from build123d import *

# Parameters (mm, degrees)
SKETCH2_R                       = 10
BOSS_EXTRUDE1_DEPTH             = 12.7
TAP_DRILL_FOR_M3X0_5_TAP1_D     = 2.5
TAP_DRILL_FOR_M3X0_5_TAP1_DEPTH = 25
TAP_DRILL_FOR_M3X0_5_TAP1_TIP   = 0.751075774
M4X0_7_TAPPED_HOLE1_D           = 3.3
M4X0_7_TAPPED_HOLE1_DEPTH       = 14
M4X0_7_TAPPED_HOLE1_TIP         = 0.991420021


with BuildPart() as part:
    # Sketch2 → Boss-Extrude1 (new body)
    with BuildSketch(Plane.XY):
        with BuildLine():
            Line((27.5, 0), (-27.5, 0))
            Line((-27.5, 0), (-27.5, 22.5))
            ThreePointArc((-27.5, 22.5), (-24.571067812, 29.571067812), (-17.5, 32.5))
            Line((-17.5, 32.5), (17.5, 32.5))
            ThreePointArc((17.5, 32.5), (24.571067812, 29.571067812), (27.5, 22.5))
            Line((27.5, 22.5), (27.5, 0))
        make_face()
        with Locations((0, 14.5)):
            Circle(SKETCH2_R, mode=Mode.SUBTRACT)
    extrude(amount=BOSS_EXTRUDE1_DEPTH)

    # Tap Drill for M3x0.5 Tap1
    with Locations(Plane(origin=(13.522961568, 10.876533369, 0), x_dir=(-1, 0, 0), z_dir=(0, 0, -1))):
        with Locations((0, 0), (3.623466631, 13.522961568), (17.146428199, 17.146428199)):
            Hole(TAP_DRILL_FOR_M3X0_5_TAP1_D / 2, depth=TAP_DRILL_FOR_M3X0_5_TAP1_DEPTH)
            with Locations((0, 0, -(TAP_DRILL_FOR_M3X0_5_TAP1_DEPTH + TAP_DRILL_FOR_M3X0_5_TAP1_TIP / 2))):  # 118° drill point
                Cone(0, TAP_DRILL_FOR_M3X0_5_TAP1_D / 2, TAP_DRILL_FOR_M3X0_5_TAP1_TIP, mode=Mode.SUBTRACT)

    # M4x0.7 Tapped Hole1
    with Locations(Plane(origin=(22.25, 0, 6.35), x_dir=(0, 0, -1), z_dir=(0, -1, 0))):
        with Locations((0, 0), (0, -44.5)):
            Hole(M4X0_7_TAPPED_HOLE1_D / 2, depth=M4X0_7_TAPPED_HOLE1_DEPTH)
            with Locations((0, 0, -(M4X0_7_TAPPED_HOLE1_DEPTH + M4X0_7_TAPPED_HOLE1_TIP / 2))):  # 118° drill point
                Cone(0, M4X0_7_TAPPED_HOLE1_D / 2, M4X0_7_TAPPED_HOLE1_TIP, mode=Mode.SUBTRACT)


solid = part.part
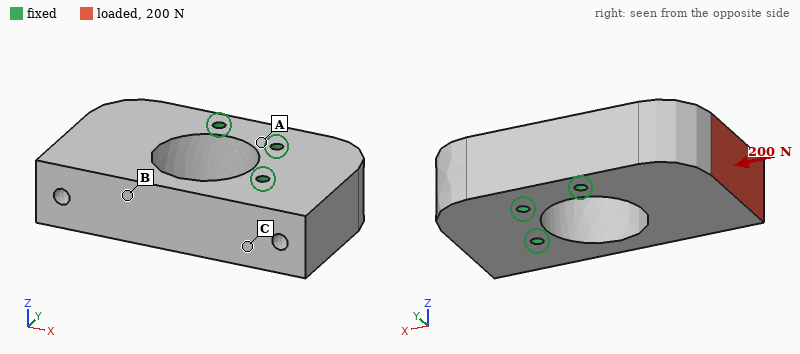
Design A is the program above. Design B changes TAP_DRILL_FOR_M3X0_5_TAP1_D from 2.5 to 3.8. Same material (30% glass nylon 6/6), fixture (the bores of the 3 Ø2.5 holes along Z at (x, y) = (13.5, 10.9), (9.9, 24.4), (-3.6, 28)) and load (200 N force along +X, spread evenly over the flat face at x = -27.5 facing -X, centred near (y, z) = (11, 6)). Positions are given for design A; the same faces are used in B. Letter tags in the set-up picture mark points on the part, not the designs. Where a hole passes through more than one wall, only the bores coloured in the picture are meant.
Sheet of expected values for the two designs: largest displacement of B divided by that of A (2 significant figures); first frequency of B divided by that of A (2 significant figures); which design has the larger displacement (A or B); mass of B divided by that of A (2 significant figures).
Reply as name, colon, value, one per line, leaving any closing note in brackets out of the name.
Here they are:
largest displacement of B divided by that of A: 0.91
first frequency of B divided by that of A: 1.1
which design has the larger displacement: A
mass of B divided by that of A: 0.99
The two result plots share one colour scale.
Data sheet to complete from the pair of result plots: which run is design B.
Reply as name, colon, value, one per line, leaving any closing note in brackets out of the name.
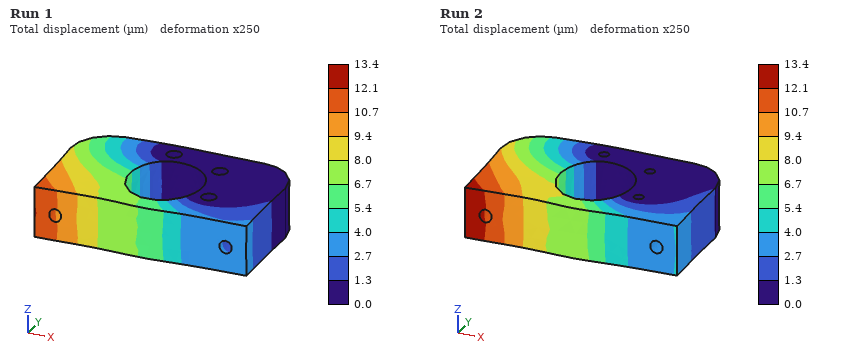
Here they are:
which run is design B: Run 1
